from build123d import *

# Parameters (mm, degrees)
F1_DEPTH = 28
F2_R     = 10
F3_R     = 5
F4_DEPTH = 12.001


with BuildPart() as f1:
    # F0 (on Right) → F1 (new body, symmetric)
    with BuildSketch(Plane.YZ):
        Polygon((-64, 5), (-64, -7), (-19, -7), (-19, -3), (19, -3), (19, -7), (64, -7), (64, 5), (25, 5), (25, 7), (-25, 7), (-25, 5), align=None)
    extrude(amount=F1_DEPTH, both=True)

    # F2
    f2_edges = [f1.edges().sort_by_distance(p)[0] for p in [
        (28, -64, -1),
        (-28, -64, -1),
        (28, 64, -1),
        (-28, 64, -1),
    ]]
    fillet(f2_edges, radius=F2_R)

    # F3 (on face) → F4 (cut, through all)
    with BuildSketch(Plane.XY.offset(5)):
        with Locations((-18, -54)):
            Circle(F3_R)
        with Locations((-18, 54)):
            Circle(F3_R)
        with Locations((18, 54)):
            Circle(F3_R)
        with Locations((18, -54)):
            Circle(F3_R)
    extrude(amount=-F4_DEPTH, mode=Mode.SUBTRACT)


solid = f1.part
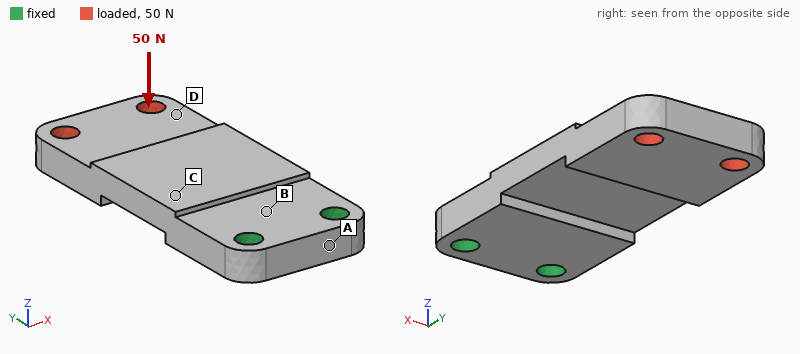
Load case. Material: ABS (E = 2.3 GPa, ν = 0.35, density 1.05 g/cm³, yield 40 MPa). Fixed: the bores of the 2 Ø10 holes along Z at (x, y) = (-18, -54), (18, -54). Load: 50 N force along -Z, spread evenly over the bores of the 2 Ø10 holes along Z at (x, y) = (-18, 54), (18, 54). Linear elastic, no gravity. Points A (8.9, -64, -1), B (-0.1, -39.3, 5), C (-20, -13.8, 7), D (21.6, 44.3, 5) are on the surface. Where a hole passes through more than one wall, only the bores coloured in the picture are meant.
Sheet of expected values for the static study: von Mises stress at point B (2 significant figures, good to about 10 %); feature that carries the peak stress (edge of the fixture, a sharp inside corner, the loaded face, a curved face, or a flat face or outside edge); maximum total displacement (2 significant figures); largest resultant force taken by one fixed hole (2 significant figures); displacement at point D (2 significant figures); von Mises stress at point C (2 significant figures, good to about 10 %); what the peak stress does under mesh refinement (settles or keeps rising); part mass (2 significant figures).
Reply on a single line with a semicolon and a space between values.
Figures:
2.8 MPa; edge of the fixture; 1.5 mm; 25 N; 1.1 mm; 3.3 MPa; keeps rising; 82 g
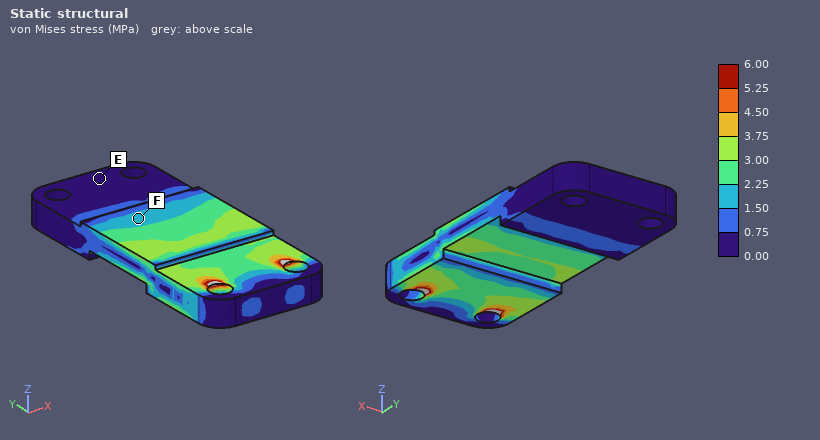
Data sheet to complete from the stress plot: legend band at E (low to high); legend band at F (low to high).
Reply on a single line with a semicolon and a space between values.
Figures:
0.00 to 0.75 MPa; 1.50 to 2.25 MPa
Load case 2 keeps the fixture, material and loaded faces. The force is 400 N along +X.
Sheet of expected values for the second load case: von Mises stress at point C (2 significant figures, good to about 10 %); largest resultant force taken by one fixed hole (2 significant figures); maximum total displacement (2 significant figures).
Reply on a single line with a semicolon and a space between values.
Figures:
2.7 MPa; 1.1 kN; 0.69 mm
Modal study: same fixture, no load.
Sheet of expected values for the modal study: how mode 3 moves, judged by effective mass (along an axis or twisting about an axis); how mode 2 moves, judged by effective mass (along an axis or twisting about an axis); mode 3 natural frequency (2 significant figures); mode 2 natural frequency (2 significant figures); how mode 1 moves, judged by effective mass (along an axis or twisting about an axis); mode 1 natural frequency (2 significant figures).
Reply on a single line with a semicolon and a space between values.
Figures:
along X; along X; 910 Hz; 760 Hz; along Z; 210 Hz
